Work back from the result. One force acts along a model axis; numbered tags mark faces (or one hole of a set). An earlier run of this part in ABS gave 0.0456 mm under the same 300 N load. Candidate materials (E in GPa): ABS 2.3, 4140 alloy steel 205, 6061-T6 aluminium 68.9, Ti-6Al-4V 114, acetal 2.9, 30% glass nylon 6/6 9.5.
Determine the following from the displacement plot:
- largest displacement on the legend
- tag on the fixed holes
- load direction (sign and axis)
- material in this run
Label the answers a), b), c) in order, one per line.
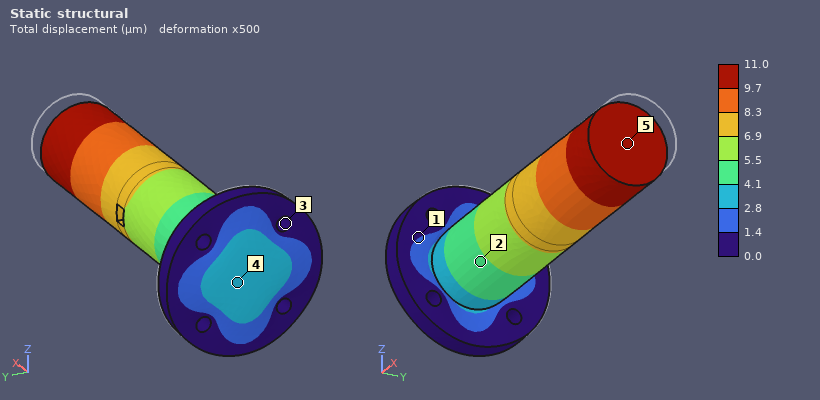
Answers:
a) 11.0 µm
b) 3
c) -X
d) 30% glass nylon 6/6
